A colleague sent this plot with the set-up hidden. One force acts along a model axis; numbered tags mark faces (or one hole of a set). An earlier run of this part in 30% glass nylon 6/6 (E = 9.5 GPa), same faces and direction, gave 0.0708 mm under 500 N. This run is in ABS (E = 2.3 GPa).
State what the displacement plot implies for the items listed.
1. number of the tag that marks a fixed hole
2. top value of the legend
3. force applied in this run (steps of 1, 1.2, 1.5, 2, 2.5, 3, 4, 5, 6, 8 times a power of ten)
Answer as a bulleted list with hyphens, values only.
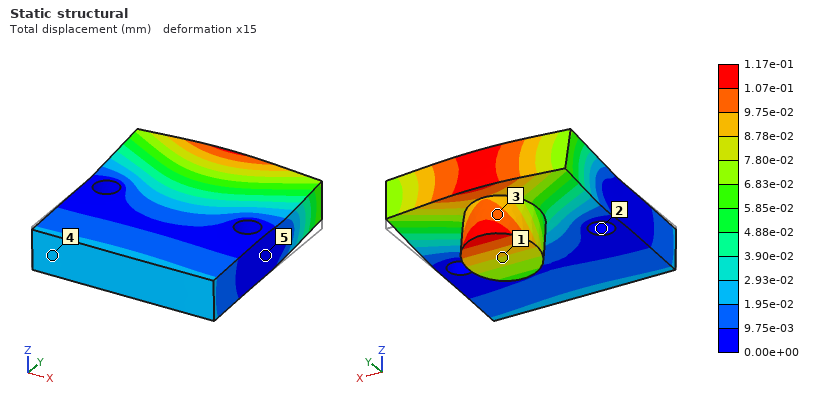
- 2
- 1.17e-01 mm
- 200 N
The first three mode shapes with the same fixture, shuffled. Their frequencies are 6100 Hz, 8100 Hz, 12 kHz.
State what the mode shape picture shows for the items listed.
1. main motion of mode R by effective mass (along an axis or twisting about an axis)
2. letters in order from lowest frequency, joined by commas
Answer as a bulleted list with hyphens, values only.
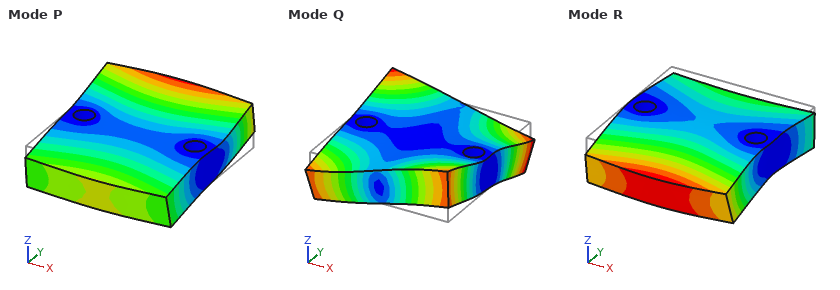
- along Z
- P, R, Q
